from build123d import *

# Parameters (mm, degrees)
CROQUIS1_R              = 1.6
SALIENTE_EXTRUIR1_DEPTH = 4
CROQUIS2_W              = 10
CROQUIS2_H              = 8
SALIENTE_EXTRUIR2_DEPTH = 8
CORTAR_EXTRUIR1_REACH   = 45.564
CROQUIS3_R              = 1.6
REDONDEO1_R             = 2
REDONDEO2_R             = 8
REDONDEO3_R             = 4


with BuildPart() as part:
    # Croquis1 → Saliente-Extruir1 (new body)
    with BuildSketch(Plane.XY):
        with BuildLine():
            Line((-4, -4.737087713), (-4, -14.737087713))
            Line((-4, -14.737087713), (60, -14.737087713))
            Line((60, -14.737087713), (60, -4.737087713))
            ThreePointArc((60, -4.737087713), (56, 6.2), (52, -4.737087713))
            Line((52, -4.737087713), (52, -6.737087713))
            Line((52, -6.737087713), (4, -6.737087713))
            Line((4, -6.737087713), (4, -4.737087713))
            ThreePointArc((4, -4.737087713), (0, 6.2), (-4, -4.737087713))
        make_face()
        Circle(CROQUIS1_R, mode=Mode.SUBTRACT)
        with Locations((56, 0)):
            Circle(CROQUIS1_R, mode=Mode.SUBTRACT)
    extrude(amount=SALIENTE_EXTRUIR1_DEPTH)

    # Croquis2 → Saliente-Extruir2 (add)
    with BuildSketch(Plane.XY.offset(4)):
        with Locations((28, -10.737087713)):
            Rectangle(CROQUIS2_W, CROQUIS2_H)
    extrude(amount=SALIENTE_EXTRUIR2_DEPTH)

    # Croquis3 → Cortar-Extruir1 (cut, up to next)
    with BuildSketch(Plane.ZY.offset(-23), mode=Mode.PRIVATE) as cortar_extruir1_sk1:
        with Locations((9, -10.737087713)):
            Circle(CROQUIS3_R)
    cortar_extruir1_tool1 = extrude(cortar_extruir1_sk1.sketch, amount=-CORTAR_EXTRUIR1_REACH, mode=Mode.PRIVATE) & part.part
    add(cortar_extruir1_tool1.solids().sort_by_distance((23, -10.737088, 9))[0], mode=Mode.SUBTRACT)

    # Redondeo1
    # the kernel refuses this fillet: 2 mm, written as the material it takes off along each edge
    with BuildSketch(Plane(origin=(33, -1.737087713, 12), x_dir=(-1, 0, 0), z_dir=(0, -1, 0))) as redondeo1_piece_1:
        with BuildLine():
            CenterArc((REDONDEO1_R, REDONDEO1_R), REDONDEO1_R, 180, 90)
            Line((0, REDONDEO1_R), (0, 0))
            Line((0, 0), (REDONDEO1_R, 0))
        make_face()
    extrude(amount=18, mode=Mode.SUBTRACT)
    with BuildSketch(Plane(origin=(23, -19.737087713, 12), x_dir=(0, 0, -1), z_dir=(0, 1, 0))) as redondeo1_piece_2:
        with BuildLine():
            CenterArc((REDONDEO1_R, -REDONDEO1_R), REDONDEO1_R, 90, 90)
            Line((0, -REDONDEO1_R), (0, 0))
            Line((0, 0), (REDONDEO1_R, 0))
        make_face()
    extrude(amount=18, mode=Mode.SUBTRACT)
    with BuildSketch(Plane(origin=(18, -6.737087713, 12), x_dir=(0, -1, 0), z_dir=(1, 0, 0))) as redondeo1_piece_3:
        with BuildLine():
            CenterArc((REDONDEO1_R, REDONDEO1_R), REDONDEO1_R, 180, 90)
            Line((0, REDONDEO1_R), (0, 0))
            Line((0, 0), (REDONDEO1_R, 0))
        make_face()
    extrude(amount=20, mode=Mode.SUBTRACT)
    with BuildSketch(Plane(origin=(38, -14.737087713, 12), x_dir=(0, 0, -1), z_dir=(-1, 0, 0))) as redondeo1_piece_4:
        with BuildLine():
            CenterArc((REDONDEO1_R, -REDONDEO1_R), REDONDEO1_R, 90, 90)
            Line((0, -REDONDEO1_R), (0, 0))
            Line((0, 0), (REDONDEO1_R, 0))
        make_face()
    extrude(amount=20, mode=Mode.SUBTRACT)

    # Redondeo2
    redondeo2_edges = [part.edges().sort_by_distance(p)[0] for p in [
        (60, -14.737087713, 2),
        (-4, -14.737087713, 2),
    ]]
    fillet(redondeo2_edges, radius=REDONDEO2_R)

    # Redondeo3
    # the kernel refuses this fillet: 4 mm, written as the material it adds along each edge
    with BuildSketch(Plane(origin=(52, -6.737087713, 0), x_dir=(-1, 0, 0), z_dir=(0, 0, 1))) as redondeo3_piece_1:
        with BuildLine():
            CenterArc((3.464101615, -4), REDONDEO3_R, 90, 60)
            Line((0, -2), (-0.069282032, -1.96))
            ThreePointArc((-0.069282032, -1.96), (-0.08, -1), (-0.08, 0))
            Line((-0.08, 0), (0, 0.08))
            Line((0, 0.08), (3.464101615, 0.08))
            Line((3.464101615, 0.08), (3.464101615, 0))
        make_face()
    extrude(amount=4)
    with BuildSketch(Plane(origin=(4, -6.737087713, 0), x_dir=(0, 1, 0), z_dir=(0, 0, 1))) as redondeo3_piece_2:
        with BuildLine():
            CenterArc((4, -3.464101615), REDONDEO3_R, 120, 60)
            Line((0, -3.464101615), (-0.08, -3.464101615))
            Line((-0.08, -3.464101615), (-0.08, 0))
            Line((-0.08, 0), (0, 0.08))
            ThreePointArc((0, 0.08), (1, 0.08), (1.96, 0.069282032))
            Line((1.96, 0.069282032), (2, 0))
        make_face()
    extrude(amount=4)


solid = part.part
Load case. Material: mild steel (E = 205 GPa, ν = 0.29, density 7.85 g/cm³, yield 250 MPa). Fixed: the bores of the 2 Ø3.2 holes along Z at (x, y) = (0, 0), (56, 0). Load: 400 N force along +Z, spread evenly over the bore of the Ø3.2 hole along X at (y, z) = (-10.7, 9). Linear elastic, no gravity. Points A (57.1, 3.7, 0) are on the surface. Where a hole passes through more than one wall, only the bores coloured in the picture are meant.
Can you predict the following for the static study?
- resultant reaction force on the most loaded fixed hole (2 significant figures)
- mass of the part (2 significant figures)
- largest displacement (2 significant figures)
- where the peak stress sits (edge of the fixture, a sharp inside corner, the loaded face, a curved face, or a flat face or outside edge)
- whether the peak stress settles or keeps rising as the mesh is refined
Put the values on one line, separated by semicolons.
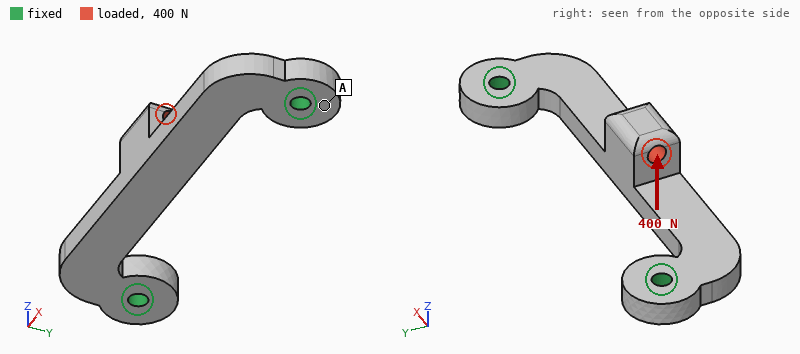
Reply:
200 N; 27 g; 57 µm; edge of the fixture; keeps rising
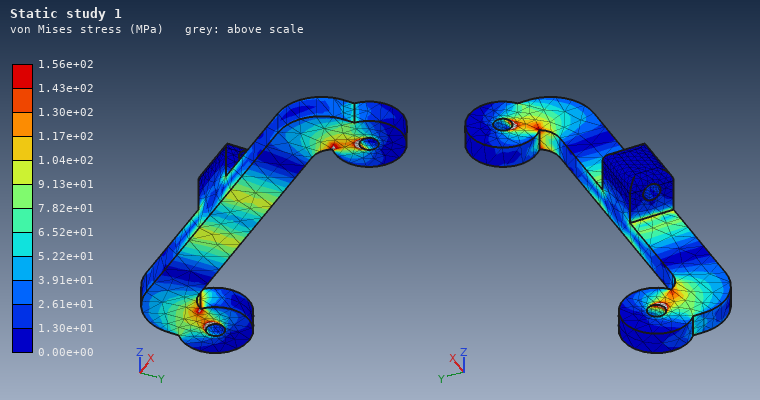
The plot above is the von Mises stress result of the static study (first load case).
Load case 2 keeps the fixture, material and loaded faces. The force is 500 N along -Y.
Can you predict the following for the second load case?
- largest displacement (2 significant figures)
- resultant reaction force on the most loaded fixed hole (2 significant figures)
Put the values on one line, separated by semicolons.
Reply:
75 µm; 400 N
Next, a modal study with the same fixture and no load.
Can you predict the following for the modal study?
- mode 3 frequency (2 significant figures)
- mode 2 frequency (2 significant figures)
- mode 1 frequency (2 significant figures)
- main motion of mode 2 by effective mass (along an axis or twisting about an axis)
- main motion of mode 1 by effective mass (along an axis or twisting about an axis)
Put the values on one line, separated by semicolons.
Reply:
10 kHz; 7400 Hz; 4100 Hz; along Y; along Z
